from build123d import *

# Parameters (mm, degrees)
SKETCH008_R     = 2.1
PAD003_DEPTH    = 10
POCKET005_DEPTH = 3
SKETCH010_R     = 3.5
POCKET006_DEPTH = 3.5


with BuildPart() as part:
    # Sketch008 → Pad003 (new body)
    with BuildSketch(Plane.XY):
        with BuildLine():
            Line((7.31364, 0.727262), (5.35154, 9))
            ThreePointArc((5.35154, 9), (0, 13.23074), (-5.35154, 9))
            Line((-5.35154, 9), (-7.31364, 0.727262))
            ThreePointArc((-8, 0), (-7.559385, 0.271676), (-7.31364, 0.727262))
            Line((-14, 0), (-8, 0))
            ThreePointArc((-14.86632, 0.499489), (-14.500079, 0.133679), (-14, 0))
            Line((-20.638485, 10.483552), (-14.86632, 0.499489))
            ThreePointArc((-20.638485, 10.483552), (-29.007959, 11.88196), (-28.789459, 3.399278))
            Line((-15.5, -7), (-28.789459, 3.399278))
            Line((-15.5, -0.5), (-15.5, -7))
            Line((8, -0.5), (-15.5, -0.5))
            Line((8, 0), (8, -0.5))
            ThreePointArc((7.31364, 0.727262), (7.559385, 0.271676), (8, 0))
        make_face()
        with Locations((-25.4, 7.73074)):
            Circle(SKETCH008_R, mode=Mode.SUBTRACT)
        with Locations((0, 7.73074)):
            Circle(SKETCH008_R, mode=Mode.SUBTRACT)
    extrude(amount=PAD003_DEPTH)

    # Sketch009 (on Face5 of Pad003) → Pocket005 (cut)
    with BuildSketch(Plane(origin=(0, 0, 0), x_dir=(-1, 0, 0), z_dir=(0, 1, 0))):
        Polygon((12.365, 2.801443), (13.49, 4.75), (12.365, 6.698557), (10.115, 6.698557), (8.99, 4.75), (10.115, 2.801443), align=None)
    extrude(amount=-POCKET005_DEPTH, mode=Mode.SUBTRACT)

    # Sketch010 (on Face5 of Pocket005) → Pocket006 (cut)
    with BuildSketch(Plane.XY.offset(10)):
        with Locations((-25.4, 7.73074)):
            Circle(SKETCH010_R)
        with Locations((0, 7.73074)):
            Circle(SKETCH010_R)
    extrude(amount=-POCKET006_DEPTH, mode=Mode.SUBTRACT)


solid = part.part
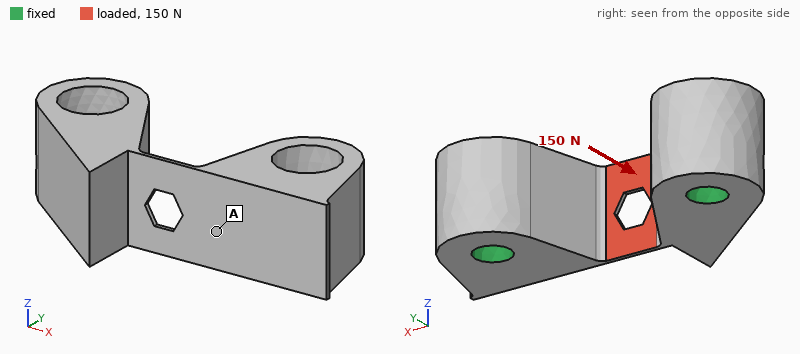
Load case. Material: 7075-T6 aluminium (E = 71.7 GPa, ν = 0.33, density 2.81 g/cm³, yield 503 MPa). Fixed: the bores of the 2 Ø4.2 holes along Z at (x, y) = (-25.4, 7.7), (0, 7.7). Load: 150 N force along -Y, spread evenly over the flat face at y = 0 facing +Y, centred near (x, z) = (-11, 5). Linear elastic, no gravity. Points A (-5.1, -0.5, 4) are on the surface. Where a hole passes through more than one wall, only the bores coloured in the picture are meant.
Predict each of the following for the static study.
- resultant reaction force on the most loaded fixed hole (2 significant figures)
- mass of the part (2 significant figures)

99 N
8.1 g
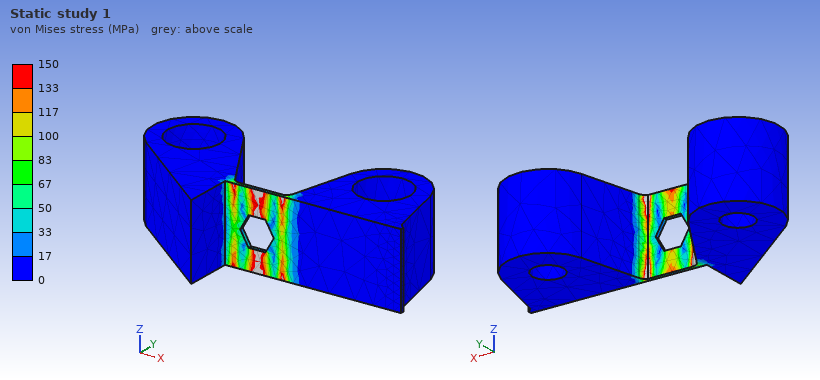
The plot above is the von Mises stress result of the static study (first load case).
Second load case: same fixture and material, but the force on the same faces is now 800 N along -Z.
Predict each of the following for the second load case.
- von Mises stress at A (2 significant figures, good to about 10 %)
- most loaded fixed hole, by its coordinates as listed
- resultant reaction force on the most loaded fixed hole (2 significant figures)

37 MPa
(0, 7.7)
440 N
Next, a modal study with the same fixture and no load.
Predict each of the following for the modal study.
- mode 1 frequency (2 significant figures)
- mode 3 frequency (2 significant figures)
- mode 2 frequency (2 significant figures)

27 kHz
44 kHz
28 kHz
